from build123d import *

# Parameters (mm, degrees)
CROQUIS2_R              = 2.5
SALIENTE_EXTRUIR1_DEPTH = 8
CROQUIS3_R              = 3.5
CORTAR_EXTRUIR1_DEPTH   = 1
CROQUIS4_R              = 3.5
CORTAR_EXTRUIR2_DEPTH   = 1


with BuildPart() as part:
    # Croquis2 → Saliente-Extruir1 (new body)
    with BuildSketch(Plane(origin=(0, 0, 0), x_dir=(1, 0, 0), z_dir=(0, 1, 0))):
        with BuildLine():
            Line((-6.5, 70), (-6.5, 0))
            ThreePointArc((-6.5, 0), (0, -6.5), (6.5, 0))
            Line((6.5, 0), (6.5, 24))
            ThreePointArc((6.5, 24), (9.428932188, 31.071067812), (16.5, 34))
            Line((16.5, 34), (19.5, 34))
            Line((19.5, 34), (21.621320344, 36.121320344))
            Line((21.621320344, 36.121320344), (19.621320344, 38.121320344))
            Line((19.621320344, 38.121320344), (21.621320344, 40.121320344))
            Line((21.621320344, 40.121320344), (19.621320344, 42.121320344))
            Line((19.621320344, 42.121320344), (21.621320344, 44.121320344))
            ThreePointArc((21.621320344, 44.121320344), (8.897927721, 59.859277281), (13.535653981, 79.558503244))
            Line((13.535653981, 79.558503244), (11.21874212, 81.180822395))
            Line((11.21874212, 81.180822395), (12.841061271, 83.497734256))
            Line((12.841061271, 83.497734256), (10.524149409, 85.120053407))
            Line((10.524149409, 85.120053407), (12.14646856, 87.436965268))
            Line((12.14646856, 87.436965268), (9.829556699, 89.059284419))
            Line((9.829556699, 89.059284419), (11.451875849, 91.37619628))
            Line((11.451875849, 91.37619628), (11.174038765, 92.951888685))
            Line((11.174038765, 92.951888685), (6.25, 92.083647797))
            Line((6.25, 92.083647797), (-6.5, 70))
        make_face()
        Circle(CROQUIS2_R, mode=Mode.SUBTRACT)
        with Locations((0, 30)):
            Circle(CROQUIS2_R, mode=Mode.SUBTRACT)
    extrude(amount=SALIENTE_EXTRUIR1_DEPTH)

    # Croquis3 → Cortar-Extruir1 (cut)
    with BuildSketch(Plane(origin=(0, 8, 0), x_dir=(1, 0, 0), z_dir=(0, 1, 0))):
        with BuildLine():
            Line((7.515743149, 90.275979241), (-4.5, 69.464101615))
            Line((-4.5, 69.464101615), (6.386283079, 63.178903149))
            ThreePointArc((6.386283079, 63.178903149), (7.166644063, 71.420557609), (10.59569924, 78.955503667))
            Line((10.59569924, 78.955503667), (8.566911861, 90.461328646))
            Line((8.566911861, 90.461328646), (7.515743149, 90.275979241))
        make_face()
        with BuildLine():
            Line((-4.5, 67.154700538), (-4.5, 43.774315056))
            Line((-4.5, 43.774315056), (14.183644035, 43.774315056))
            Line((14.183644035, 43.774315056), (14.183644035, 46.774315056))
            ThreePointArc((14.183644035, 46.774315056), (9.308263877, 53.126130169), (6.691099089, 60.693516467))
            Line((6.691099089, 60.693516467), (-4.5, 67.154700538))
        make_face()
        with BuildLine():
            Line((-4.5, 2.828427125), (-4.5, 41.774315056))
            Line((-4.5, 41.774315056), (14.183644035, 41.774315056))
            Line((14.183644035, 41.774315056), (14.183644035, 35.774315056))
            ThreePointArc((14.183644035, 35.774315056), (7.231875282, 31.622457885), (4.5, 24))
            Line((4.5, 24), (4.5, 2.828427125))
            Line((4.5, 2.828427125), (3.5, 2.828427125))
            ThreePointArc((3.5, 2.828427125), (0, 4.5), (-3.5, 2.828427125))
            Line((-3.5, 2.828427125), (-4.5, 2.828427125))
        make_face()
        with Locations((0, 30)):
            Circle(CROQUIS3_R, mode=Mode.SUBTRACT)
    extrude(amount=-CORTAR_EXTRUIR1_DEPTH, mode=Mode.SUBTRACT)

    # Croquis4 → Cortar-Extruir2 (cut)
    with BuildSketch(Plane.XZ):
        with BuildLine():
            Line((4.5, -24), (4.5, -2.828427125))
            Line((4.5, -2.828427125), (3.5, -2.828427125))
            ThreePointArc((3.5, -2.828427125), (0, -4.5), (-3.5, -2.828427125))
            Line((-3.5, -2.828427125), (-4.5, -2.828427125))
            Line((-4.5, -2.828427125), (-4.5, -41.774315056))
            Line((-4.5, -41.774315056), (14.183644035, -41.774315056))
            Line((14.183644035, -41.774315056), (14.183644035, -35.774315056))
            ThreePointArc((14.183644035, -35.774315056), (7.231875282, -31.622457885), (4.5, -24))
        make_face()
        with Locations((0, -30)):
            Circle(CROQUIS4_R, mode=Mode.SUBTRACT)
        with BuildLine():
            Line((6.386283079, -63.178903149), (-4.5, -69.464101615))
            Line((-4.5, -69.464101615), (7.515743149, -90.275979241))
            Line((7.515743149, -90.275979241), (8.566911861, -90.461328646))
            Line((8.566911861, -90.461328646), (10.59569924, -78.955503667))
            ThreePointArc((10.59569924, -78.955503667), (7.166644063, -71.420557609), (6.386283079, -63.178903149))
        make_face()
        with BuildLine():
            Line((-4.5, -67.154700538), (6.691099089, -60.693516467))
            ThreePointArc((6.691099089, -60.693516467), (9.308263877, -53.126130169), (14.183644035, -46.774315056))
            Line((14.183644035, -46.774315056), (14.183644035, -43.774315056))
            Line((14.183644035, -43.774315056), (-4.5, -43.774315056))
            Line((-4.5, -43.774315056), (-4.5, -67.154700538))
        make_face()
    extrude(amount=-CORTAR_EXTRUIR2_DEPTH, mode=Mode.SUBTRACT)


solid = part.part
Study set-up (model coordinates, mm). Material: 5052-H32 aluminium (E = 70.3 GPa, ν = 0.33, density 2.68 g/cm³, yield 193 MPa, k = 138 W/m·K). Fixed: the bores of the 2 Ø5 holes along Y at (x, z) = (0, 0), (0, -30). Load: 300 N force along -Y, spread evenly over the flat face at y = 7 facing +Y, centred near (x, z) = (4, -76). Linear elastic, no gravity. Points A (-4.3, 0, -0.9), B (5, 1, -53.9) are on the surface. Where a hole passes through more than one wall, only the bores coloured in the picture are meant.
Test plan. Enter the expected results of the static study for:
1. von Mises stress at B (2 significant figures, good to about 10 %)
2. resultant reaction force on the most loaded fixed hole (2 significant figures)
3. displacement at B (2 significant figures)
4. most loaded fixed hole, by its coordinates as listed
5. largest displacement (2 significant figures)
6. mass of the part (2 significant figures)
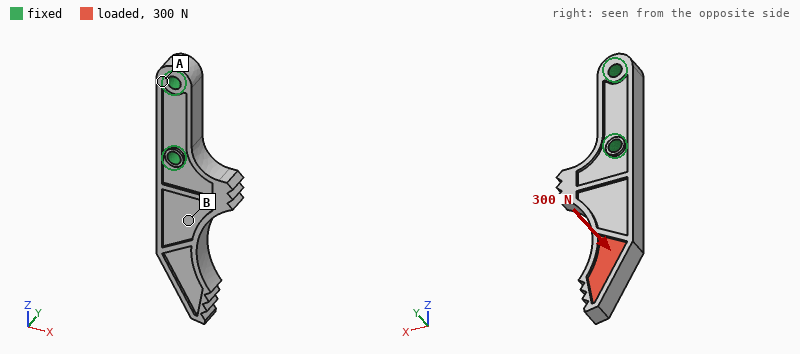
53 MPa
350 N
0.11 mm
(0, -30)
0.53 mm
27 g
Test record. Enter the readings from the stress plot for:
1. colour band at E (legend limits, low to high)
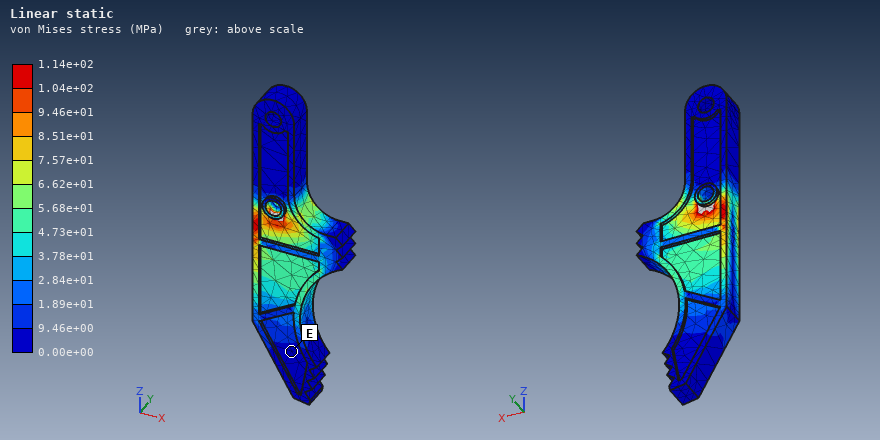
0.00e+00 to 9.46e+00 MPa
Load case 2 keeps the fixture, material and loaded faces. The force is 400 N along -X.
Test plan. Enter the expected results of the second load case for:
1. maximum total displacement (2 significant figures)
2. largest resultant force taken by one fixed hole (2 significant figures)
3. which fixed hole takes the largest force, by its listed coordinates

0.16 mm
660 N
(0, -30)
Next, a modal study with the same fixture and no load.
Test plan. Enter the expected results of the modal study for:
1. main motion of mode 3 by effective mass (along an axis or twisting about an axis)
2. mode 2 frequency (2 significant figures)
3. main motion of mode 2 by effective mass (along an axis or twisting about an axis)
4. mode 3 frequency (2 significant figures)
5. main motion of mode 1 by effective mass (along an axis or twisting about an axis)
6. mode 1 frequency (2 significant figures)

twisting about Z
3500 Hz
along X
7800 Hz
along Y
1700 Hz
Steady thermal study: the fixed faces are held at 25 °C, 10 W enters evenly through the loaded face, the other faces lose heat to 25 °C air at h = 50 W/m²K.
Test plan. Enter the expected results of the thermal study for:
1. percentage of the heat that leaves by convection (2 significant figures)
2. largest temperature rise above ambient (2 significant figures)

23 %
26 K
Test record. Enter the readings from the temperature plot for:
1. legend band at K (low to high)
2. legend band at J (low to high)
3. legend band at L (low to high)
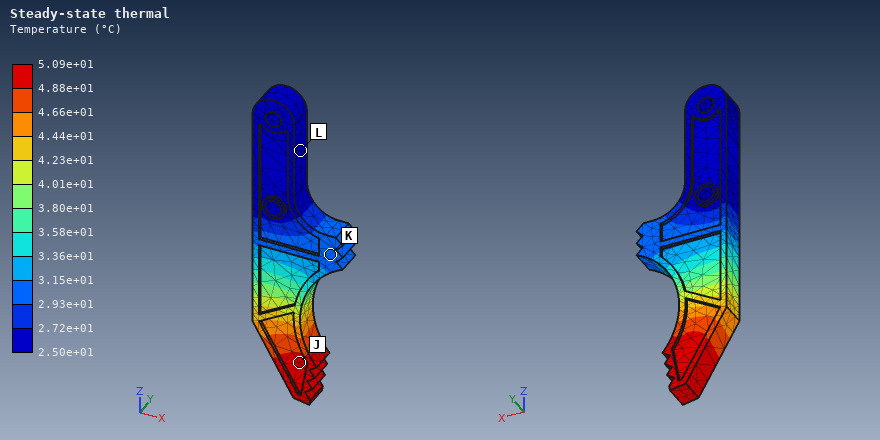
2.93e+01 to 3.15e+01 °C
4.88e+01 to 5.09e+01 °C
2.50e+01 to 2.72e+01 °C
